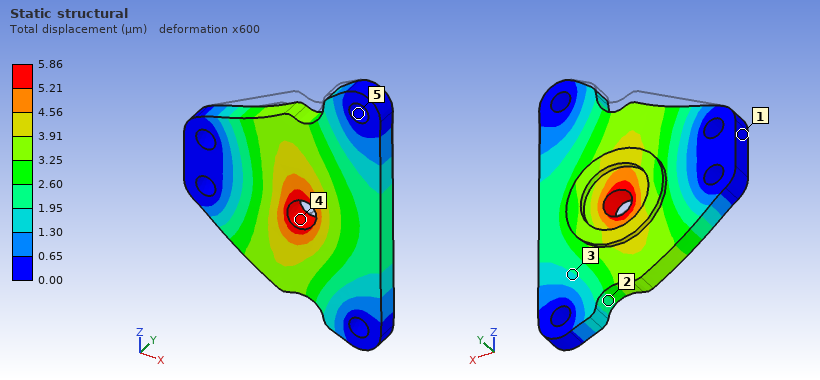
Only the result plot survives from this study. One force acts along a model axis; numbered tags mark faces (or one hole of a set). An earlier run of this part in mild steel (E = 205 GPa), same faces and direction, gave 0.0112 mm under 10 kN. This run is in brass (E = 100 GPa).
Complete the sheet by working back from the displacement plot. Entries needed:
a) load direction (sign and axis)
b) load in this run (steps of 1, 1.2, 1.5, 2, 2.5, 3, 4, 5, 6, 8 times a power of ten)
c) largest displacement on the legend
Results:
-Z
2.5 kN
5.86 µm
